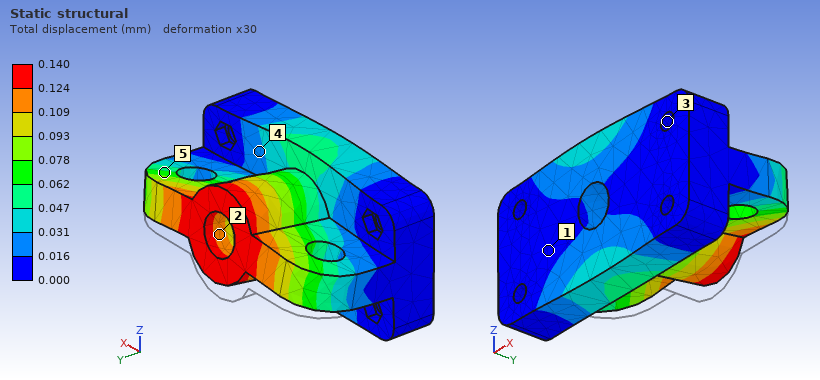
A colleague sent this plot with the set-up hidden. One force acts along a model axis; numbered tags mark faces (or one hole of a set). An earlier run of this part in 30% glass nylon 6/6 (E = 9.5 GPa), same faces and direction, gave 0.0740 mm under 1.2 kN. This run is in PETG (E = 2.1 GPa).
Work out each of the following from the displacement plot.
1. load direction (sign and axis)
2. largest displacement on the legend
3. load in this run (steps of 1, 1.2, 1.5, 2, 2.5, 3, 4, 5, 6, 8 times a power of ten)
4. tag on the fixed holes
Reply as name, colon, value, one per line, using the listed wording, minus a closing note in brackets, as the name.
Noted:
load direction: +Z
largest displacement on the legend: 0.140 mm
load in this run: 500 N
tag on the fixed holes: 3
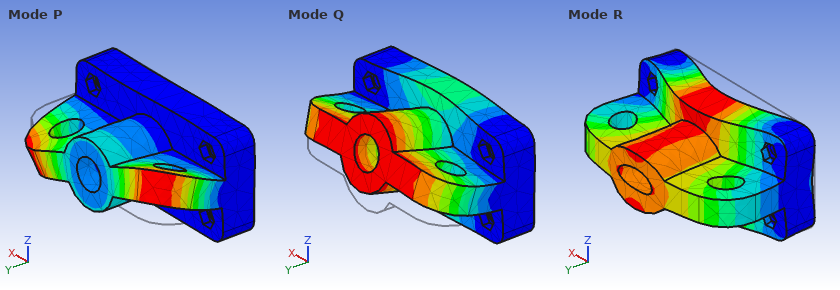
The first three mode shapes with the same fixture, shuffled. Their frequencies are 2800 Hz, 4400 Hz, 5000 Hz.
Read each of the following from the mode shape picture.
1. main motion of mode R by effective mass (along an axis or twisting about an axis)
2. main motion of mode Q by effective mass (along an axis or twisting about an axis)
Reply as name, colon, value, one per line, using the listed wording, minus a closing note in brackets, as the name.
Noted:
main motion of mode R by effective mass: along Y
main motion of mode Q by effective mass: along Z
